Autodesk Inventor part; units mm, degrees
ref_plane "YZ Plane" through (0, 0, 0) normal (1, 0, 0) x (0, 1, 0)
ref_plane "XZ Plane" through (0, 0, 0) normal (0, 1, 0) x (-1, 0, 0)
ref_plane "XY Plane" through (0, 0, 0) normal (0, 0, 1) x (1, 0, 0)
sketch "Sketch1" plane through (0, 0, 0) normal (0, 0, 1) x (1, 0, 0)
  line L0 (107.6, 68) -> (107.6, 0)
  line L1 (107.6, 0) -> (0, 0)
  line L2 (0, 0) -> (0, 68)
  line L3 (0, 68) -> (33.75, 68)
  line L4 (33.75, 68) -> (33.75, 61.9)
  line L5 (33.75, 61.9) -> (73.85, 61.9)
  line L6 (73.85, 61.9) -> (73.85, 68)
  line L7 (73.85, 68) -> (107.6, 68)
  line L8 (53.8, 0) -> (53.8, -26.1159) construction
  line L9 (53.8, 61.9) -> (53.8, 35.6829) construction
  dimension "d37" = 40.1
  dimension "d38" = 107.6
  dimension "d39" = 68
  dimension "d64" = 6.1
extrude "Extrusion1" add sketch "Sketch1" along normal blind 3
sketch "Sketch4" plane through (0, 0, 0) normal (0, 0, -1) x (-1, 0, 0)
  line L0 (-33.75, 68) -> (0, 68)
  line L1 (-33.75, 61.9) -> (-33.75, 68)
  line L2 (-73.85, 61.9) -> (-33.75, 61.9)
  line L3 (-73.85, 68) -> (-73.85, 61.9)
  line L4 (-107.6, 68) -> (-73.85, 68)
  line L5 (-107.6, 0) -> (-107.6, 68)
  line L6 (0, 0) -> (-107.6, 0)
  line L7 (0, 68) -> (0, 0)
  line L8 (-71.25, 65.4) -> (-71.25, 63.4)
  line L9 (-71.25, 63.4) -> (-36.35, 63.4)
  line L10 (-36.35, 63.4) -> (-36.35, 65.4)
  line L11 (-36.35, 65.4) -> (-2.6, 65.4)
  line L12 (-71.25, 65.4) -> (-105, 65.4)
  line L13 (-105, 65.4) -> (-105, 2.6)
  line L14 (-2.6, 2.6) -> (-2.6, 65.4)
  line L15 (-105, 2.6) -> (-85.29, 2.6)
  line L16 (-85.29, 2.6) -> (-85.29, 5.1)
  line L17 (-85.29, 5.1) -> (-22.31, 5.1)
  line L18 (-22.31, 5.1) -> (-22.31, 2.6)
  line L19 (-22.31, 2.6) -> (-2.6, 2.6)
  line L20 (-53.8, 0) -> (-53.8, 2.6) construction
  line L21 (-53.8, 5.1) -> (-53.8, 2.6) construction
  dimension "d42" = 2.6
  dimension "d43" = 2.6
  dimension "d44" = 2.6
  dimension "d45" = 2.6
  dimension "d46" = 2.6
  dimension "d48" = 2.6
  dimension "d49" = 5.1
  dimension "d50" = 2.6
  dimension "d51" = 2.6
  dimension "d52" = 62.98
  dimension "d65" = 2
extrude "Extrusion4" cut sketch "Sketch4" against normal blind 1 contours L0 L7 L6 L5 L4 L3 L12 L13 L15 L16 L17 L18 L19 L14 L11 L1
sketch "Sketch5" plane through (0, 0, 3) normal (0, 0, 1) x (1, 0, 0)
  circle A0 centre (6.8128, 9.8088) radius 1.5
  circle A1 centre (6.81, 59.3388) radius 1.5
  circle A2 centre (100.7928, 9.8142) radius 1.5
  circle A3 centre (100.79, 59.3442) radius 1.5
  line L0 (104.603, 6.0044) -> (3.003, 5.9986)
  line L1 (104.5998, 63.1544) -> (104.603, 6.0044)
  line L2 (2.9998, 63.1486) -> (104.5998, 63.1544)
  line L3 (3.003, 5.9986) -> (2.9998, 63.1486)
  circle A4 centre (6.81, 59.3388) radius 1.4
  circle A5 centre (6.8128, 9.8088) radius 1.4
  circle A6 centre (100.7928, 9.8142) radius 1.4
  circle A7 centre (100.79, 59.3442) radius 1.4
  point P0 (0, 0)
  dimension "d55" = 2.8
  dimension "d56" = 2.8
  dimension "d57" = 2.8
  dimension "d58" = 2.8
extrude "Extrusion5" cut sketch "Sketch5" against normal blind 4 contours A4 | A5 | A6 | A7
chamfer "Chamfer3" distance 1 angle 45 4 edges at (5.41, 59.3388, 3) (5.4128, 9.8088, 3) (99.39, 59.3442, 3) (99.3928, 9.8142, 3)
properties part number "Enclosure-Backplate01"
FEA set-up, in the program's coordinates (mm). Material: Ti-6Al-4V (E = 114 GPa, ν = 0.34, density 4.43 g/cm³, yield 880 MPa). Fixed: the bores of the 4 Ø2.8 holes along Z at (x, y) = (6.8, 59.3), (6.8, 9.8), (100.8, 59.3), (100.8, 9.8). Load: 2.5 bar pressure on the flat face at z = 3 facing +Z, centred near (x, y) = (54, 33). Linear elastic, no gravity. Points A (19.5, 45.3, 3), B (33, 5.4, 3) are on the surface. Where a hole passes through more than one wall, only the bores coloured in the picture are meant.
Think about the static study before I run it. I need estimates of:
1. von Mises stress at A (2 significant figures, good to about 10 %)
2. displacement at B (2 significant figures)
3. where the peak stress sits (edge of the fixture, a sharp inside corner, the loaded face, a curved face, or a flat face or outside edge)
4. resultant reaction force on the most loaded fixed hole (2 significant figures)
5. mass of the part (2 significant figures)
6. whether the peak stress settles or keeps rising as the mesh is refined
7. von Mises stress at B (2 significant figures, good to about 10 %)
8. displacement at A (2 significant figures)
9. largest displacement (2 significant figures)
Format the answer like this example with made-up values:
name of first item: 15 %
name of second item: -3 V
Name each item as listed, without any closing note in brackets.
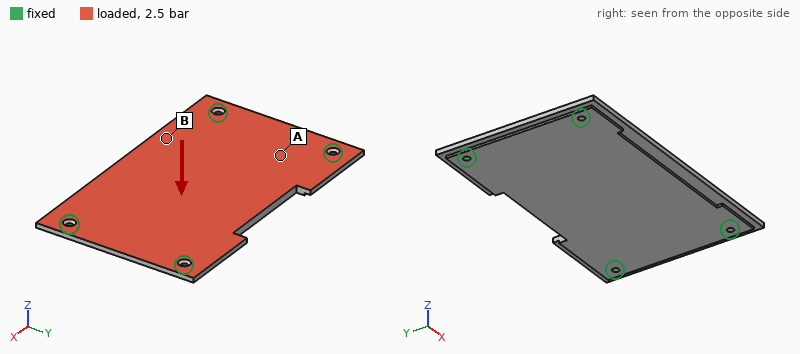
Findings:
von Mises stress at A: 26 MPa
displacement at B: 0.22 mm
where the peak stress sits: edge of the fixture
resultant reaction force on the most loaded fixed hole: 590 N
mass of the part: 89 g
whether the peak stress settles or keeps rising as the mesh is refined: keeps rising
von Mises stress at B: 52 MPa
displacement at A: 0.12 mm
largest displacement: 0.34 mm
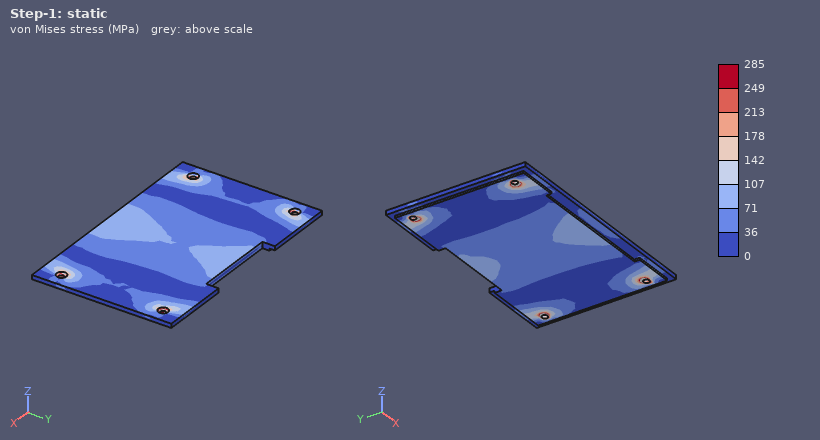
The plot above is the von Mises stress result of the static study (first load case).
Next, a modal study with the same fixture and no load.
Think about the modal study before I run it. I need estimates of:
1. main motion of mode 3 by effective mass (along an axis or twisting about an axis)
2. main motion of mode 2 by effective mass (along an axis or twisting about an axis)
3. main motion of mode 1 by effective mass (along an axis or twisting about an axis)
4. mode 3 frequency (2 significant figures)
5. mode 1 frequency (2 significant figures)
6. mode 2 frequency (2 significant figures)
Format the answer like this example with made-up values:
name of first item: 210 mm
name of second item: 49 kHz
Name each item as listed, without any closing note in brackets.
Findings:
main motion of mode 3 by effective mass: twisting about Y
main motion of mode 2 by effective mass: twisting about X
main motion of mode 1 by effective mass: along Z
mode 3 frequency: 3800 Hz
mode 1 frequency: 1400 Hz
mode 2 frequency: 2400 Hz
